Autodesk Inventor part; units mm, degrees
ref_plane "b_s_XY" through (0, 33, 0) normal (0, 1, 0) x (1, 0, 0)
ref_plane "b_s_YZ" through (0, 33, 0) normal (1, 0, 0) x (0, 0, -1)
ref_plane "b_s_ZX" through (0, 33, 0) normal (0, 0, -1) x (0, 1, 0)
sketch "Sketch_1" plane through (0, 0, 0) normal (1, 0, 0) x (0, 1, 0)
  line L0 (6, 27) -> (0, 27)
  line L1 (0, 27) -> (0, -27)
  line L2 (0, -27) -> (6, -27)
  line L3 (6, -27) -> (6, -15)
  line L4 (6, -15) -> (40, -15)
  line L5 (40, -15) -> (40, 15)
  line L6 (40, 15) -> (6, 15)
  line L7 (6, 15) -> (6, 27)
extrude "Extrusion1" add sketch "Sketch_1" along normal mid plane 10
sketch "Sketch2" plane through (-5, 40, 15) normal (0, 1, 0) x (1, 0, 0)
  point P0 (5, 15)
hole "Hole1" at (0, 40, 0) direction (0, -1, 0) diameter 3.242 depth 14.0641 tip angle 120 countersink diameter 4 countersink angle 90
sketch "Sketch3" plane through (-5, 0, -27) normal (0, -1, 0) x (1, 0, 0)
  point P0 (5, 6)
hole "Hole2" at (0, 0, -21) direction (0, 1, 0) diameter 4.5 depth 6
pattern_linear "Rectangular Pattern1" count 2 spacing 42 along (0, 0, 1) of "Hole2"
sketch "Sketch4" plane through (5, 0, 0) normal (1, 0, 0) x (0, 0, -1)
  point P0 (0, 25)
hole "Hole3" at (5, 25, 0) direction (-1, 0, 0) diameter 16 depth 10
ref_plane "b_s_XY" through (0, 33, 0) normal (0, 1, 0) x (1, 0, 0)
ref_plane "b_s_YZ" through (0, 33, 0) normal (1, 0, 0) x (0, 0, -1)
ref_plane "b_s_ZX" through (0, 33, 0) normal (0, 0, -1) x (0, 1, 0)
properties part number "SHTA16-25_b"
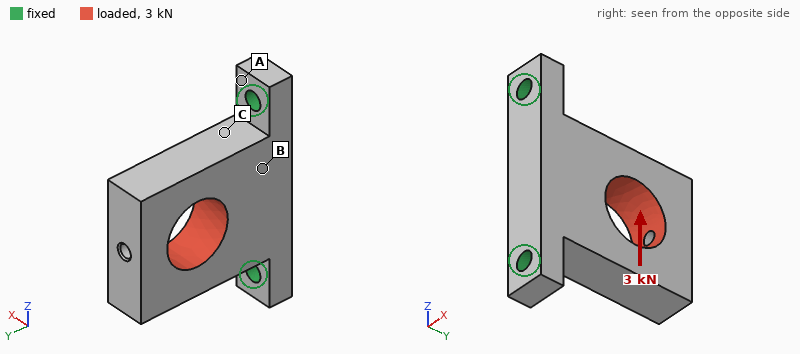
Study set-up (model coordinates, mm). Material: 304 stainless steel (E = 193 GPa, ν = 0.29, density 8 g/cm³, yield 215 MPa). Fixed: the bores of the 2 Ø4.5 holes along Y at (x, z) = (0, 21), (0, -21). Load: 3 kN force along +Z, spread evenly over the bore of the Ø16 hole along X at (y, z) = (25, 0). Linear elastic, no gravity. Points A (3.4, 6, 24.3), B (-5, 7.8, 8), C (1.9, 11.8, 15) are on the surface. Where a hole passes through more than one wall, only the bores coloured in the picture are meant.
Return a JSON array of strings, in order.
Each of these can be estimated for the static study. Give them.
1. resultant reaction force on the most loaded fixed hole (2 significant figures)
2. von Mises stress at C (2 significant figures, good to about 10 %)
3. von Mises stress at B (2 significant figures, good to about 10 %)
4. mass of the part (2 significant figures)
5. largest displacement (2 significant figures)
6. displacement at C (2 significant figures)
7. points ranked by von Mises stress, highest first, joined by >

["2.4 kN", "44 MPa", "24 MPa", "89 g", "26 µm", "7.4 µm", "C > B > A"]
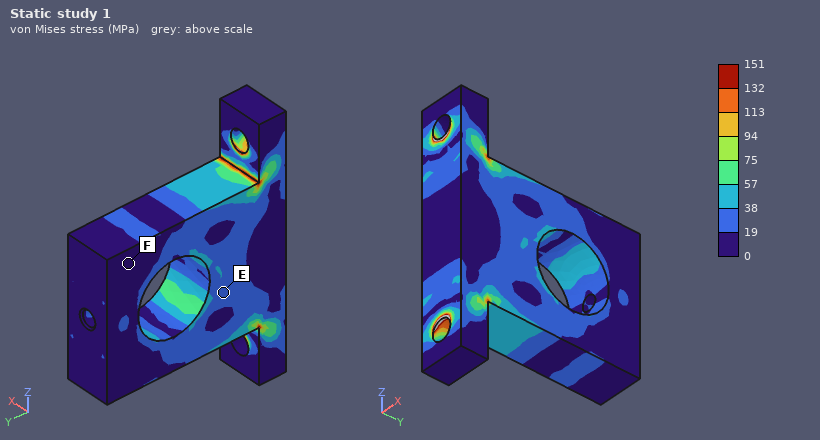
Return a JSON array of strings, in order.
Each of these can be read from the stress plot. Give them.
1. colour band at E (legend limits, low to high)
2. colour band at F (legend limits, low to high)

["19 to 38 MPa", "0 to 19 MPa"]
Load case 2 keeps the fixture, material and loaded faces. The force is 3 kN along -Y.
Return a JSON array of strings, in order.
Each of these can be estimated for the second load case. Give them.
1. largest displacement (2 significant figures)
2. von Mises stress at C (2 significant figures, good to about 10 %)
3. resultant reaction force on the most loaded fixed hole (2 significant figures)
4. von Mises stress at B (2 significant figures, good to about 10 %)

["7.3 µm", "25 MPa", "1.6 kN", "13 MPa"]
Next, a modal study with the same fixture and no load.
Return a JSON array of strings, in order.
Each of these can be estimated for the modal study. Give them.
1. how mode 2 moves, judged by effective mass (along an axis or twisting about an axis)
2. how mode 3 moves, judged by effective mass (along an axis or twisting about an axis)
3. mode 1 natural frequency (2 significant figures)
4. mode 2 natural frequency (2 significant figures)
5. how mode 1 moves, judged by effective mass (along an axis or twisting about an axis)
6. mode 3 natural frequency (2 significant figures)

["along Z", "twisting about Y", "2600 Hz", "8200 Hz", "along X", "9900 Hz"]
